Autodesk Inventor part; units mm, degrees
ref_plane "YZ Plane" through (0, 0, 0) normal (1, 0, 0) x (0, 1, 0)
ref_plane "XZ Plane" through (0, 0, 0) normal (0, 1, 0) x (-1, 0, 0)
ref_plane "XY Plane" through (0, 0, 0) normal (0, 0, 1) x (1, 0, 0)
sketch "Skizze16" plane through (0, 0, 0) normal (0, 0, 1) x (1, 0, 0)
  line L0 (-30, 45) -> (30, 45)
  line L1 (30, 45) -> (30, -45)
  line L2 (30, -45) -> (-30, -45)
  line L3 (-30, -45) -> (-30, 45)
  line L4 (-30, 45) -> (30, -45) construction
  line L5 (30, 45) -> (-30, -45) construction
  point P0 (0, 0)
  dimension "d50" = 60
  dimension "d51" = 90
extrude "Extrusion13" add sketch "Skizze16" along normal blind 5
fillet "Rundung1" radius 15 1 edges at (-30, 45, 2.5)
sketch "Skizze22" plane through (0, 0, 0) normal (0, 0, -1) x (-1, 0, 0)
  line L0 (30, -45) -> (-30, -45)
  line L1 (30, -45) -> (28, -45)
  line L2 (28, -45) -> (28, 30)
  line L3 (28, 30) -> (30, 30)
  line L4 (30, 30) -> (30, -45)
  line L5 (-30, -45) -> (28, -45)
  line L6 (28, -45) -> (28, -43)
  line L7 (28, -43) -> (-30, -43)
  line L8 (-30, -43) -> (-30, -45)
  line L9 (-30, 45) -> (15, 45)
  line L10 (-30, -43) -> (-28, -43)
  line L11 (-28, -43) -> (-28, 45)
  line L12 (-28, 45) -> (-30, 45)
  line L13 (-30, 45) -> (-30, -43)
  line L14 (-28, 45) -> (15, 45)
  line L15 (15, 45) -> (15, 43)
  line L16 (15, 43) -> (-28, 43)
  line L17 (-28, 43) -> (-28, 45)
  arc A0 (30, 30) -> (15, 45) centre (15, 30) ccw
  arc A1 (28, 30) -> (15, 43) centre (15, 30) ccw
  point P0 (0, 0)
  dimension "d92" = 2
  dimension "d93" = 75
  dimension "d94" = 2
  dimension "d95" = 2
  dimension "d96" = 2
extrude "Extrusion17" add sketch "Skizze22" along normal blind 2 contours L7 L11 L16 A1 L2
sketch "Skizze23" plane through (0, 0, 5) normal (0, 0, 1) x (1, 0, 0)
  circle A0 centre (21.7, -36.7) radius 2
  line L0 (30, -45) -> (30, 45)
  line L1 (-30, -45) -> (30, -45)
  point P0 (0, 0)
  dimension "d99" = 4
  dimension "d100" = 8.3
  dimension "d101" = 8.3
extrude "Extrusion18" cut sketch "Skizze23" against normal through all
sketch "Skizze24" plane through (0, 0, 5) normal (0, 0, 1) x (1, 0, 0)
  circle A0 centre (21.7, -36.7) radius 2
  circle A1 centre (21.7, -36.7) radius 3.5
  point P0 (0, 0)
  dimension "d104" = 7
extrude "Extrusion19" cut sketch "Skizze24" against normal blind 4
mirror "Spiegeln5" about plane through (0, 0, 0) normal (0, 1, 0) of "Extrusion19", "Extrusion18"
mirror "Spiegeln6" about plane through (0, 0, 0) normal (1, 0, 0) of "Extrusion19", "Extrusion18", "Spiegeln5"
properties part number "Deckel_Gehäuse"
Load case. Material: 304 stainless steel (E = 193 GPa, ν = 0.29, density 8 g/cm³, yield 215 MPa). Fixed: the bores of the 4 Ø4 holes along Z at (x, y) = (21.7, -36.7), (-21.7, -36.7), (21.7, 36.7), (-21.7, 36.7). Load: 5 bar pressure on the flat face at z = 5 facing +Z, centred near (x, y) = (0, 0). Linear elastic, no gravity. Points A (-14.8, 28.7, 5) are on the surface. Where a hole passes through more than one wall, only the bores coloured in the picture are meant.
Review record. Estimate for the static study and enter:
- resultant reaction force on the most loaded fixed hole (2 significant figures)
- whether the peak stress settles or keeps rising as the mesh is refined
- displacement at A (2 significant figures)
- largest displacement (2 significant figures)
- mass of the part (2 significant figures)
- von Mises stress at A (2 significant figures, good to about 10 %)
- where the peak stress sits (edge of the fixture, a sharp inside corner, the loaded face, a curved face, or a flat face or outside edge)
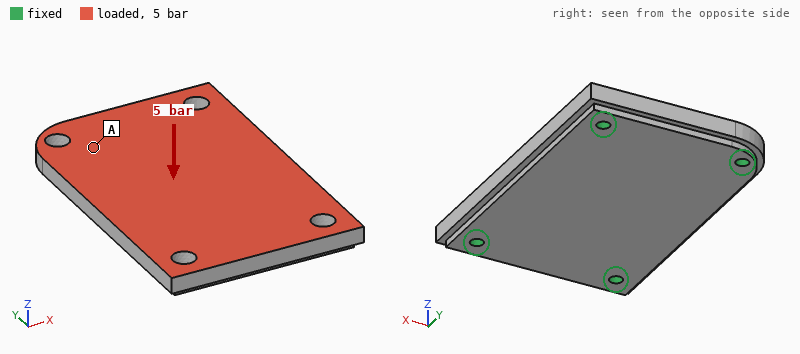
970 N
keeps rising
6.0 µm
16 µm
280 g
10 MPa
edge of the fixture
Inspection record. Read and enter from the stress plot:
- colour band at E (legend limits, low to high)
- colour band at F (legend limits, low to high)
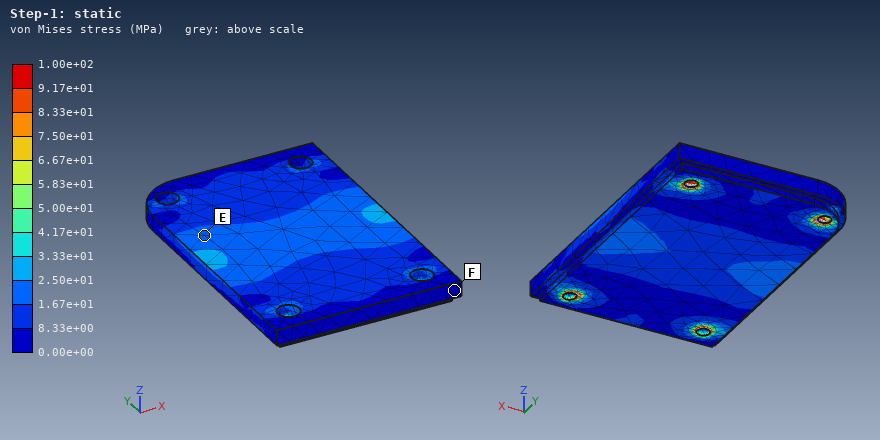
1.67e+01 to 2.50e+01 MPa
0.00e+00 to 8.33e+00 MPa
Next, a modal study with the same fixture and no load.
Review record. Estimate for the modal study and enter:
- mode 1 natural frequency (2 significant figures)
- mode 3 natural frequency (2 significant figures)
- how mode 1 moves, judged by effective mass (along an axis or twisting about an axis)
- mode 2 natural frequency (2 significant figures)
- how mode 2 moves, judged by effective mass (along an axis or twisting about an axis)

4200 Hz
11 kHz
along Z
6600 Hz
twisting about Y
